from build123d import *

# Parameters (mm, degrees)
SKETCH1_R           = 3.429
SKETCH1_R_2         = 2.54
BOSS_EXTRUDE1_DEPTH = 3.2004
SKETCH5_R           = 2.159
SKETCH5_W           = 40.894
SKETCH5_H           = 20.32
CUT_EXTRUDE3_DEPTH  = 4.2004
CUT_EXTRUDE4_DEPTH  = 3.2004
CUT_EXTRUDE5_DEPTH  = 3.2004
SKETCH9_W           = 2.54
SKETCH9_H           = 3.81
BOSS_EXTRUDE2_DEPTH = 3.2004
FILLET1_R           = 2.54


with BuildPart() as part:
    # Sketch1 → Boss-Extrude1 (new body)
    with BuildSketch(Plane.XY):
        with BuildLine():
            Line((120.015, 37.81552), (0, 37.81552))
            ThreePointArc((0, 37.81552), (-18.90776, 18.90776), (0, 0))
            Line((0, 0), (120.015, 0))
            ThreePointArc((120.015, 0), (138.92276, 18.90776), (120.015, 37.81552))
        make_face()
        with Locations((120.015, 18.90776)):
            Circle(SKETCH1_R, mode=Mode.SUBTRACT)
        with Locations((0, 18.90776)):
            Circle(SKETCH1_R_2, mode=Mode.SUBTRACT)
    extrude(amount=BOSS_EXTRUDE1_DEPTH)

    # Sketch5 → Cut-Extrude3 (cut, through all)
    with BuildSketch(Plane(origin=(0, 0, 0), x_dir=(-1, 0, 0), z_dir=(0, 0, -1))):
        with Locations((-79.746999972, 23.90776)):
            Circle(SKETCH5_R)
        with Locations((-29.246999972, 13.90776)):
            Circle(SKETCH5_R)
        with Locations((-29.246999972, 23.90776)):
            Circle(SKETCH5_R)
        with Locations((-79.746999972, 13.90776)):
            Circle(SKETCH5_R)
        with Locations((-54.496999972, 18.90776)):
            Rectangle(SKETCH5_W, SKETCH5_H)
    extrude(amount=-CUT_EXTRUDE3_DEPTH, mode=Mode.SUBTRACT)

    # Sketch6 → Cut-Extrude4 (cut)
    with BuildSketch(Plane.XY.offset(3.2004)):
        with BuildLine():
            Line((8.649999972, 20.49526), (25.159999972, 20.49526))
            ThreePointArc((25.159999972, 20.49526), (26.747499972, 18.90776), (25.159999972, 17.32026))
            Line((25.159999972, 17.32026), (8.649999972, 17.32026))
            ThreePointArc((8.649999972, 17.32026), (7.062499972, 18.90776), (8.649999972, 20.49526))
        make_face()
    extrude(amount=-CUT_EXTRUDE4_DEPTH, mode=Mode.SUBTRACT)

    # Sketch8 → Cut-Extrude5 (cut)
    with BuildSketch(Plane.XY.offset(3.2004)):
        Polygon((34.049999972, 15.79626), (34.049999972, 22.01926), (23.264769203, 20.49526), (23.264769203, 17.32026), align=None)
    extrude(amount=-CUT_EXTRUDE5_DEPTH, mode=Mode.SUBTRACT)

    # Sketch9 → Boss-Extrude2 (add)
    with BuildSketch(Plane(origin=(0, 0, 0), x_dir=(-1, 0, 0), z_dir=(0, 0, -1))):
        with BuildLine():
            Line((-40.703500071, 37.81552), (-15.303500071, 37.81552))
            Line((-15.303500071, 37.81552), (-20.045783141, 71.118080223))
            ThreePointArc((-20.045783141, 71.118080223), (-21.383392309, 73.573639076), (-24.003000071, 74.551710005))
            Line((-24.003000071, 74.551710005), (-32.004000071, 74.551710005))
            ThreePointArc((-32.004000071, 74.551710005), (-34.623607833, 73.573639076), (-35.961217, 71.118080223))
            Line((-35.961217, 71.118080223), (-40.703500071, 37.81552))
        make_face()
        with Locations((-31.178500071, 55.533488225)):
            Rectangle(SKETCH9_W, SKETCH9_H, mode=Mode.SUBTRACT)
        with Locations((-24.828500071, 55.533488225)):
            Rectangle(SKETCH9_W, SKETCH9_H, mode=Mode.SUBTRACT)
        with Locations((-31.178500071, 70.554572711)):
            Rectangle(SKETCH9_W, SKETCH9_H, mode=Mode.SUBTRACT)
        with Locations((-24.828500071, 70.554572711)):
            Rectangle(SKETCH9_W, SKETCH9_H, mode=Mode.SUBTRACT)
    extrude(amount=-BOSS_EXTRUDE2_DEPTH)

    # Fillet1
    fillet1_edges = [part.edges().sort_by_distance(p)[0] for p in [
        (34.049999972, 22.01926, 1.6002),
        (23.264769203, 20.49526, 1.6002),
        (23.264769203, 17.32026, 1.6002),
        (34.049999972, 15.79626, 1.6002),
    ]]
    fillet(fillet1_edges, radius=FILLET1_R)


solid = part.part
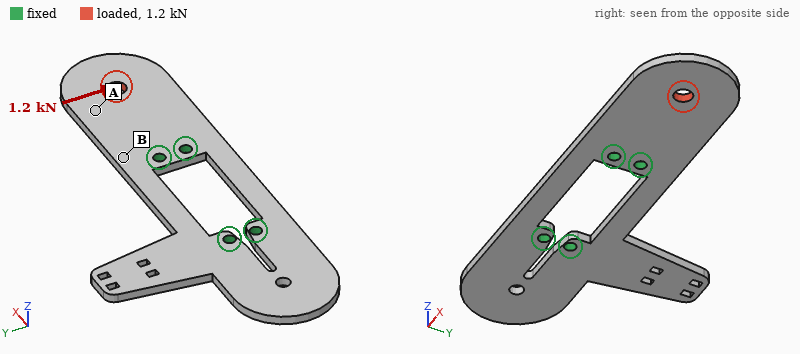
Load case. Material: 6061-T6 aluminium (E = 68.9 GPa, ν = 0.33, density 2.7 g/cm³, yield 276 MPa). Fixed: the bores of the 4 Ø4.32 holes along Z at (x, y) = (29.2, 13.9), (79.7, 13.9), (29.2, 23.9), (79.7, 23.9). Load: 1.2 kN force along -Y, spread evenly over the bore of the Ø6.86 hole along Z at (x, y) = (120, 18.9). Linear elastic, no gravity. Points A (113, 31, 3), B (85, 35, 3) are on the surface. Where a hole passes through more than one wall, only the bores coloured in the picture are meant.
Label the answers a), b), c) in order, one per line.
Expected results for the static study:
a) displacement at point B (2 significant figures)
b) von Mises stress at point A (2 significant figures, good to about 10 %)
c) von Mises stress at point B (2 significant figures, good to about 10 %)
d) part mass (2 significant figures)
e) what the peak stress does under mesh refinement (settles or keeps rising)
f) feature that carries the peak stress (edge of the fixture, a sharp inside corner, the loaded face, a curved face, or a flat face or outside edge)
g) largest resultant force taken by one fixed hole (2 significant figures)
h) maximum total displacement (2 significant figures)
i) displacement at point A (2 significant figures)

a) 0.023 mm
b) 17 MPa
c) 35 MPa
d) 46 g
e) keeps rising
f) edge of the fixture
g) 2.3 kN
h) 0.12 mm
i) 0.071 mm
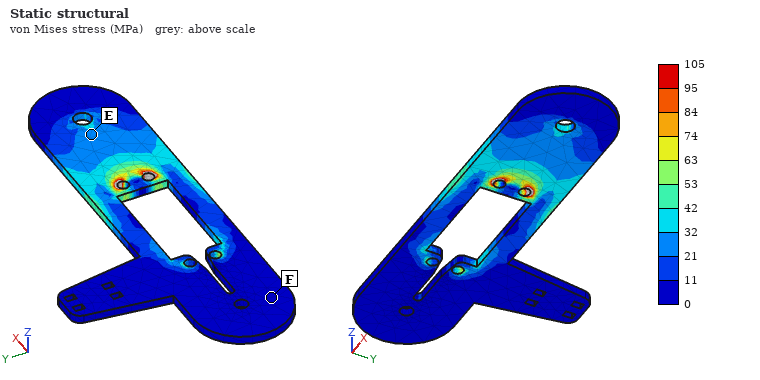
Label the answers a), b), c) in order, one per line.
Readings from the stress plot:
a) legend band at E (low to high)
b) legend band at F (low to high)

a) 21 to 32 MPa
b) 0 to 11 MPa
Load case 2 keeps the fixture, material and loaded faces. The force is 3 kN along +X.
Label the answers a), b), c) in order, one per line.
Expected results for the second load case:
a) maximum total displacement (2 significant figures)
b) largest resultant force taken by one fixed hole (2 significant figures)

a) 24 µm
b) 1.4 kN
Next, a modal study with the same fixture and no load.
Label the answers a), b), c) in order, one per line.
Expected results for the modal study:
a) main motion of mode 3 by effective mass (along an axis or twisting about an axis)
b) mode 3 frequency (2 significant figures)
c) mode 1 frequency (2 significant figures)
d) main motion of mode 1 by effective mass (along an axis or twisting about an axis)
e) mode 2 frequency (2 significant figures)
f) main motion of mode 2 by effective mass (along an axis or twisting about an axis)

a) along Z
b) 1300 Hz
c) 880 Hz
d) along Z
e) 1300 Hz
f) twisting about X
